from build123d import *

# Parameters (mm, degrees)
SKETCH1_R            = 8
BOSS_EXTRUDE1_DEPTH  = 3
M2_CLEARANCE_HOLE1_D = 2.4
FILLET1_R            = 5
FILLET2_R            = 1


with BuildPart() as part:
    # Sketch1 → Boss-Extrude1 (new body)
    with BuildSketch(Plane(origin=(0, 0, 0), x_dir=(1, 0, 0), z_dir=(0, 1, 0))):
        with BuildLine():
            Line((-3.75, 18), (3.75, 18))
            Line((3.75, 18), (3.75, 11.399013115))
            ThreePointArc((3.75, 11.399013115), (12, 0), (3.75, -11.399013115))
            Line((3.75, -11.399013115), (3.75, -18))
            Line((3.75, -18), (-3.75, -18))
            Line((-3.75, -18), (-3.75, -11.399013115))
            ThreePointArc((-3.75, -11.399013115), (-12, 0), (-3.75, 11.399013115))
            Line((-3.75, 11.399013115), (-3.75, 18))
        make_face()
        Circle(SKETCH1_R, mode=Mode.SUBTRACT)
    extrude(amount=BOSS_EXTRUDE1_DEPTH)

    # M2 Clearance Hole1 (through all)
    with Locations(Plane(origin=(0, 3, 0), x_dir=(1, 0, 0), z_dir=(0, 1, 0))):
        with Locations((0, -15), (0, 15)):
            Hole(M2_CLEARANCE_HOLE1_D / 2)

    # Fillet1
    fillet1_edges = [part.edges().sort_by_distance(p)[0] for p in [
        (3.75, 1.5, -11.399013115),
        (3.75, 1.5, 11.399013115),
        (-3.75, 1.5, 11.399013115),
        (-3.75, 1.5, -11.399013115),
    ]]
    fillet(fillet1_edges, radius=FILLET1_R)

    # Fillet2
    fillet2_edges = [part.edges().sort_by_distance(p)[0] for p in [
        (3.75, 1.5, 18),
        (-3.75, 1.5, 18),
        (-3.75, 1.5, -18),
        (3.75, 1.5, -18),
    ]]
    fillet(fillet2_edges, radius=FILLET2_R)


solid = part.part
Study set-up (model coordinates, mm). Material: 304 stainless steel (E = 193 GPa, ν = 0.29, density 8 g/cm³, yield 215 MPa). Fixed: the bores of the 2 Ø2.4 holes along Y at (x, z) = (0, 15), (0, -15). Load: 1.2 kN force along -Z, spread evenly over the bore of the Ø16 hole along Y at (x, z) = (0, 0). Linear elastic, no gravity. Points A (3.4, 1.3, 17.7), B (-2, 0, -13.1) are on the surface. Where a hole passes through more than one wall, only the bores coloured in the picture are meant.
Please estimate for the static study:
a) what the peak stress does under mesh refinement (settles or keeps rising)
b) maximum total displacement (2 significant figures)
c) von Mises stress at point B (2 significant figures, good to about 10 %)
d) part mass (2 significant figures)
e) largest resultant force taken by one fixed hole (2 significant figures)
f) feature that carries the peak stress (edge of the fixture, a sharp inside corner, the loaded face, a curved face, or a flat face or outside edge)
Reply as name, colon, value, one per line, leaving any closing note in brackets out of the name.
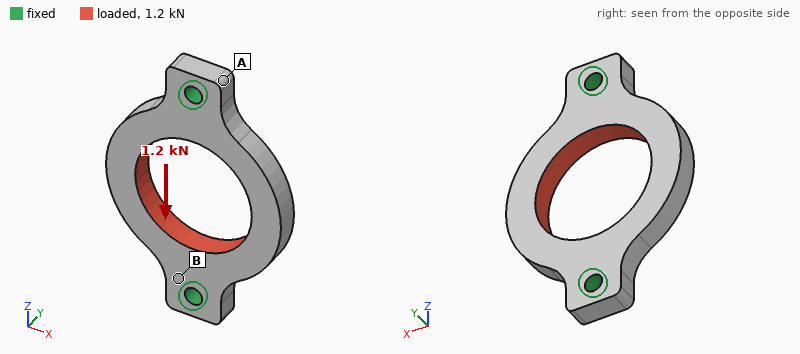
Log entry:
what the peak stress does under mesh refinement: keeps rising
maximum total displacement: 3.2 µm
von Mises stress at point B: 29 MPa
part mass: 8.2 g
largest resultant force taken by one fixed hole: 600 N
feature that carries the peak stress: edge of the fixture
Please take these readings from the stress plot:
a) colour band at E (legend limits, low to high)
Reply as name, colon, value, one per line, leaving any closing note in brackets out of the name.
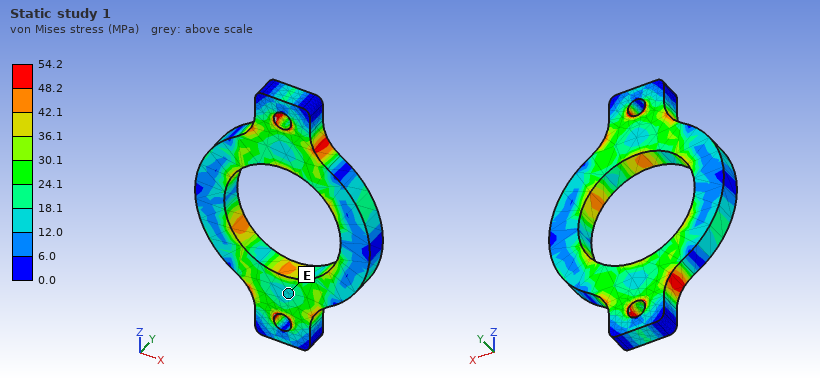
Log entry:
colour band at E: 12.0 to 18.1 MPa
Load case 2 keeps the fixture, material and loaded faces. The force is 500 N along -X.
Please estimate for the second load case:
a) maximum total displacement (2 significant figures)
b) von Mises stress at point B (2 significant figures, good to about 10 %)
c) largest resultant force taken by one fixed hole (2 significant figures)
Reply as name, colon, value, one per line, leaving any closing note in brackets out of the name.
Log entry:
maximum total displacement: 1.5 µm
von Mises stress at point B: 20 MPa
largest resultant force taken by one fixed hole: 250 N
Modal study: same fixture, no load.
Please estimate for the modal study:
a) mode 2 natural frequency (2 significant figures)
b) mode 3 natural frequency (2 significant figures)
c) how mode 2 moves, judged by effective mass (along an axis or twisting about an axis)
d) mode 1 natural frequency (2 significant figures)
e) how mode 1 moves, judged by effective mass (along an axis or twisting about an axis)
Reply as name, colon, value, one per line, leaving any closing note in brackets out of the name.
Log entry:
mode 2 natural frequency: 11 kHz
mode 3 natural frequency: 28 kHz
how mode 2 moves, judged by effective mass: along Y
mode 1 natural frequency: 9800 Hz
how mode 1 moves, judged by effective mass: twisting about Z
